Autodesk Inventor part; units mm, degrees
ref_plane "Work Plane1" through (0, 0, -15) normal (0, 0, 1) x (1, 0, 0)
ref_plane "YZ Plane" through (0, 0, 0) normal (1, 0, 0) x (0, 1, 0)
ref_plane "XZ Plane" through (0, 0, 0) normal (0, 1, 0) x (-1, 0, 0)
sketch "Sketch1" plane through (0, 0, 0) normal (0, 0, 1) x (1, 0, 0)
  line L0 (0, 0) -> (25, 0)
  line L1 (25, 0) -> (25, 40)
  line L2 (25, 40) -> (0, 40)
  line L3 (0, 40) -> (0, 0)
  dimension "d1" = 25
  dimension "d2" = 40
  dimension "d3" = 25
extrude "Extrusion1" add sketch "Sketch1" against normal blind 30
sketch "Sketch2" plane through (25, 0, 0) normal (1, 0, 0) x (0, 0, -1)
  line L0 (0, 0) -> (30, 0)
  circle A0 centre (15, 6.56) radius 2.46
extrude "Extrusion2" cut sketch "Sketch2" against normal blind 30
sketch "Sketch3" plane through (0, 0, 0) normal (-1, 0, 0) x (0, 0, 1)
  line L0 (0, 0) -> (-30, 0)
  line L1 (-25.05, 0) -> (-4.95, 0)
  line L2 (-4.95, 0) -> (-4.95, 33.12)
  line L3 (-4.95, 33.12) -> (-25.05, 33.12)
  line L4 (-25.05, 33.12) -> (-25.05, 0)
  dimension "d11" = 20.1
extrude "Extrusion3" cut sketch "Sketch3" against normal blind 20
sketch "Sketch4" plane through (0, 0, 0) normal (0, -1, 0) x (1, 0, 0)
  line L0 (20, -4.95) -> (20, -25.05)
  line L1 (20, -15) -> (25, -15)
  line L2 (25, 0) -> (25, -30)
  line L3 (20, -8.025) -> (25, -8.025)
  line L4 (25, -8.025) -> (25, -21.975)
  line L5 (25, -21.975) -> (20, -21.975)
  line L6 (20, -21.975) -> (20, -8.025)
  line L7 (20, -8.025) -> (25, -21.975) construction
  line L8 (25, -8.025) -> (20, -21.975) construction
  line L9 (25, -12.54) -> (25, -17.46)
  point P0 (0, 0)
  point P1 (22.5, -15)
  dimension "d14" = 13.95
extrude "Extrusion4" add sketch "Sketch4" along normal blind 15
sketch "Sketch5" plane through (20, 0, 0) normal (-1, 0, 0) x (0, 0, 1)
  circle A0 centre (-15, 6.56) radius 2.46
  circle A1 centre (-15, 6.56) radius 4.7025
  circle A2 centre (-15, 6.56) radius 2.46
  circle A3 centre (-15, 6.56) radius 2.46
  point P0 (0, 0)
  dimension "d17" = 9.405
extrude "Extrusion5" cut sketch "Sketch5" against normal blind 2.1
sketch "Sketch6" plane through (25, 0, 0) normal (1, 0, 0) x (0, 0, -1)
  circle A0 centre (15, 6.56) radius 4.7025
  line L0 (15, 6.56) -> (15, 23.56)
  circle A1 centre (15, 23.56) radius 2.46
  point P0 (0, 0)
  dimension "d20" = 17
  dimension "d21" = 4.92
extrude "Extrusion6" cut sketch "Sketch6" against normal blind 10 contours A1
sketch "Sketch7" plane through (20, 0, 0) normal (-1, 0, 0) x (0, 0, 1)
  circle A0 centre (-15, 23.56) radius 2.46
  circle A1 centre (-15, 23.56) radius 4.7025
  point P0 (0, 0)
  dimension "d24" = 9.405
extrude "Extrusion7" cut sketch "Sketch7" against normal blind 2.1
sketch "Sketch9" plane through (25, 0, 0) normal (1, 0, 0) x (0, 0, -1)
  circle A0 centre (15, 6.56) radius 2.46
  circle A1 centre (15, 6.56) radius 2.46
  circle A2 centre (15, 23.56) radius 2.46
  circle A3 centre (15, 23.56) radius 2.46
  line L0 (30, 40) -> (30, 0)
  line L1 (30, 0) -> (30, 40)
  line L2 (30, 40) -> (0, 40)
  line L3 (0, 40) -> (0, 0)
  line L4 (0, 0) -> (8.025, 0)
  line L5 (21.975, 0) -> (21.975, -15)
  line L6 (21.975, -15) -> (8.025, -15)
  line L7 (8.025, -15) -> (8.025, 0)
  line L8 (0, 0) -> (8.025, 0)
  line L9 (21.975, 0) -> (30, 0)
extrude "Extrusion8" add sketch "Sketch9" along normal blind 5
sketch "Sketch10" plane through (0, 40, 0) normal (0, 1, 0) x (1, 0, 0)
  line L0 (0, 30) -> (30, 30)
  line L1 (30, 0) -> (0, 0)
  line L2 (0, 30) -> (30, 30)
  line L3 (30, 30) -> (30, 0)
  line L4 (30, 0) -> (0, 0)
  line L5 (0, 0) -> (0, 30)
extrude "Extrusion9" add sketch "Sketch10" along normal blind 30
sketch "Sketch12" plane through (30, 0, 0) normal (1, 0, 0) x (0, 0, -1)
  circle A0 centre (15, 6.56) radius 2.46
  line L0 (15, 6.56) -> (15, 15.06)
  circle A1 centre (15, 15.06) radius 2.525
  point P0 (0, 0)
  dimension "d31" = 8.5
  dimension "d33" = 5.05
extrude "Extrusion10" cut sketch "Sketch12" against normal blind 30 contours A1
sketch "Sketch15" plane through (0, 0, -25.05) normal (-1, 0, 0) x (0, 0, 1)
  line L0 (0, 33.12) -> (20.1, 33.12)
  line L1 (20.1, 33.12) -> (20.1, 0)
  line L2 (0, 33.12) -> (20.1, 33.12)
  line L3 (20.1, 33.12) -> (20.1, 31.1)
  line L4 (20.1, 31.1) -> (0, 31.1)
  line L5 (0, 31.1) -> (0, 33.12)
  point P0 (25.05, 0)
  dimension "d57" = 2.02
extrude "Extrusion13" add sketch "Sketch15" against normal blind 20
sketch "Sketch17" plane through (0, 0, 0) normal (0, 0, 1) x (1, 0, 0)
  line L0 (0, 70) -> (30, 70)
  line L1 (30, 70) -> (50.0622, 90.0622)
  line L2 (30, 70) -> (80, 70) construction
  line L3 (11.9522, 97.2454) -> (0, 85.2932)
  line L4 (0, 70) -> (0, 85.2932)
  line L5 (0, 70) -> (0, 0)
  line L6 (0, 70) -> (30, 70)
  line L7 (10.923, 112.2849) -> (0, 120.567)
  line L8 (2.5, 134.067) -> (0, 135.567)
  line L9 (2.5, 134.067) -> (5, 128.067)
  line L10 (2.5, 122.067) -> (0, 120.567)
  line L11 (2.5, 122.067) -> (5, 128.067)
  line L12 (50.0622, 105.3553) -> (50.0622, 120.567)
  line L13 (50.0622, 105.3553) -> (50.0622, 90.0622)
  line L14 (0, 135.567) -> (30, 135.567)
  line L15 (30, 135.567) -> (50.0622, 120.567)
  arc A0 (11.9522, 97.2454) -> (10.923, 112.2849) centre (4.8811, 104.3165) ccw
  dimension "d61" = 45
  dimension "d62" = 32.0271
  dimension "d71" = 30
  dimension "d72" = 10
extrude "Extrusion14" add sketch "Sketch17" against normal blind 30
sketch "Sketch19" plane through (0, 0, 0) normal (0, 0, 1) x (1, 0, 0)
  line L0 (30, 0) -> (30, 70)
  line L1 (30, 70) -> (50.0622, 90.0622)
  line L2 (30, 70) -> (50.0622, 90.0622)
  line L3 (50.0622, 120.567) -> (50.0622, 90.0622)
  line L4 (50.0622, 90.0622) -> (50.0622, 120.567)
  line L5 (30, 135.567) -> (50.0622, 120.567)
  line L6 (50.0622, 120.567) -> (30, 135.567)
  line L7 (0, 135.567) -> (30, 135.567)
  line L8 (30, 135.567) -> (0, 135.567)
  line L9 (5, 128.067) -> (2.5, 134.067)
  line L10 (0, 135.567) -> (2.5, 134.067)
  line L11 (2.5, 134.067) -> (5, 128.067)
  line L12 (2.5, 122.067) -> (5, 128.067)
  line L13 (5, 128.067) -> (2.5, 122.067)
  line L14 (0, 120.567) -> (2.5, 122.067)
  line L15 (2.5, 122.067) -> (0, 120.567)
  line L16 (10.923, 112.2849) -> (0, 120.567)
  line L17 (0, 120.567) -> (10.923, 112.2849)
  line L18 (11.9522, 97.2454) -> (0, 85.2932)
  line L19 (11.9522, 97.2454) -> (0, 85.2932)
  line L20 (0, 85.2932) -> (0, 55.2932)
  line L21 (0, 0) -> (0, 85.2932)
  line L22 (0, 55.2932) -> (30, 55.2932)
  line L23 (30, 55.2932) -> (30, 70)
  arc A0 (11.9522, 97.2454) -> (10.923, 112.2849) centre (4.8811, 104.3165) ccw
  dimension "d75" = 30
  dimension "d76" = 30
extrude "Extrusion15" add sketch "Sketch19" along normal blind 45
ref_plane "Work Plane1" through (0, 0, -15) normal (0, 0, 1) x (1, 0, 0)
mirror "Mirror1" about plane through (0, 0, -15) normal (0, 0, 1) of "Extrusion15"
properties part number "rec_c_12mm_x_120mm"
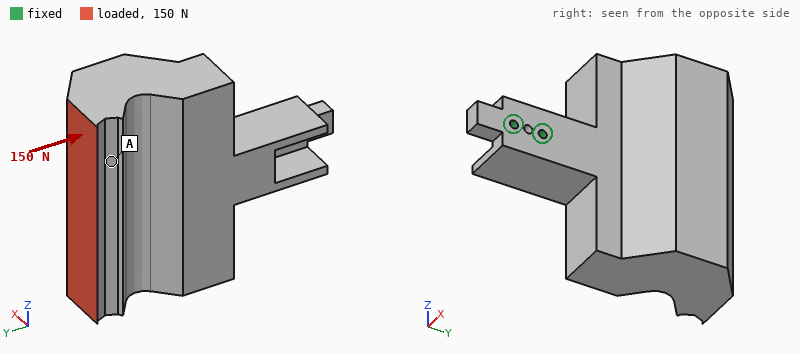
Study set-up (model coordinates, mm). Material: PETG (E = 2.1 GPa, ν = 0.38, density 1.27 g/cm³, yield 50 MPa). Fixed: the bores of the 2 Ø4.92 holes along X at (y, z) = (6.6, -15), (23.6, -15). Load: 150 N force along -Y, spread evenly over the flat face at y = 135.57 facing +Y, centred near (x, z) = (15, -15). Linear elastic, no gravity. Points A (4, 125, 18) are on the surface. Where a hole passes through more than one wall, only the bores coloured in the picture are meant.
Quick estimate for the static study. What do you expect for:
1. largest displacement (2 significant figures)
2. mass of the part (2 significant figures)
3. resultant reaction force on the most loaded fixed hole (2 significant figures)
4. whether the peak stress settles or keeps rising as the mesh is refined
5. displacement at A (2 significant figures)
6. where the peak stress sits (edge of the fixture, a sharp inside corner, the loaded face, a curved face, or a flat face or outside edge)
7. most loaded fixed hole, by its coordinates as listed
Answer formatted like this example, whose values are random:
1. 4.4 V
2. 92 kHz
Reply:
1. 0.14 mm
2. 510 g
3. 110 N
4. keeps rising
5. 0.12 mm
6. edge of the fixture
7. (23.6, -15)
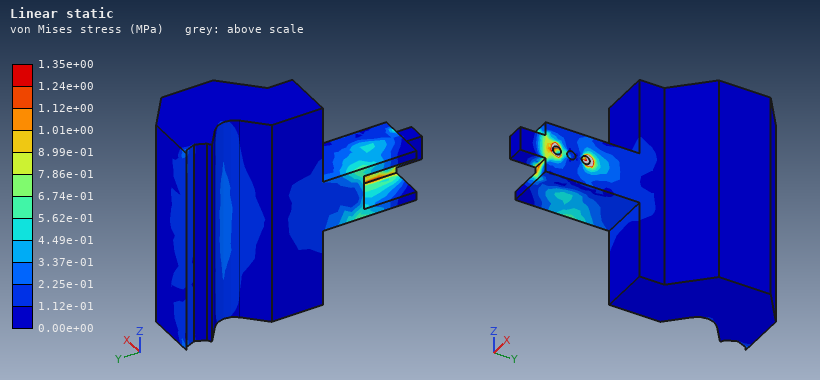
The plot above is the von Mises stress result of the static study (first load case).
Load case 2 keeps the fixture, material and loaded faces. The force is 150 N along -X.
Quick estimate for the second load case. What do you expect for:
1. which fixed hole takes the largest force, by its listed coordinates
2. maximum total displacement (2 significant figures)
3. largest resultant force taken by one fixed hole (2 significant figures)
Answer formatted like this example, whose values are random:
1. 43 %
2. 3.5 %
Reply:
1. (23.6, -15)
2. 1.8 mm
3. 820 N
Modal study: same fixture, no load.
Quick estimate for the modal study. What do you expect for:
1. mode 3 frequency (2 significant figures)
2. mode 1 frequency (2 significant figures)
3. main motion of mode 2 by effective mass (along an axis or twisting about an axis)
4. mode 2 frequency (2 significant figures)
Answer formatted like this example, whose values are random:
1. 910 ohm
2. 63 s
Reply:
1. 150 Hz
2. 100 Hz
3. along Z
4. 110 Hz
